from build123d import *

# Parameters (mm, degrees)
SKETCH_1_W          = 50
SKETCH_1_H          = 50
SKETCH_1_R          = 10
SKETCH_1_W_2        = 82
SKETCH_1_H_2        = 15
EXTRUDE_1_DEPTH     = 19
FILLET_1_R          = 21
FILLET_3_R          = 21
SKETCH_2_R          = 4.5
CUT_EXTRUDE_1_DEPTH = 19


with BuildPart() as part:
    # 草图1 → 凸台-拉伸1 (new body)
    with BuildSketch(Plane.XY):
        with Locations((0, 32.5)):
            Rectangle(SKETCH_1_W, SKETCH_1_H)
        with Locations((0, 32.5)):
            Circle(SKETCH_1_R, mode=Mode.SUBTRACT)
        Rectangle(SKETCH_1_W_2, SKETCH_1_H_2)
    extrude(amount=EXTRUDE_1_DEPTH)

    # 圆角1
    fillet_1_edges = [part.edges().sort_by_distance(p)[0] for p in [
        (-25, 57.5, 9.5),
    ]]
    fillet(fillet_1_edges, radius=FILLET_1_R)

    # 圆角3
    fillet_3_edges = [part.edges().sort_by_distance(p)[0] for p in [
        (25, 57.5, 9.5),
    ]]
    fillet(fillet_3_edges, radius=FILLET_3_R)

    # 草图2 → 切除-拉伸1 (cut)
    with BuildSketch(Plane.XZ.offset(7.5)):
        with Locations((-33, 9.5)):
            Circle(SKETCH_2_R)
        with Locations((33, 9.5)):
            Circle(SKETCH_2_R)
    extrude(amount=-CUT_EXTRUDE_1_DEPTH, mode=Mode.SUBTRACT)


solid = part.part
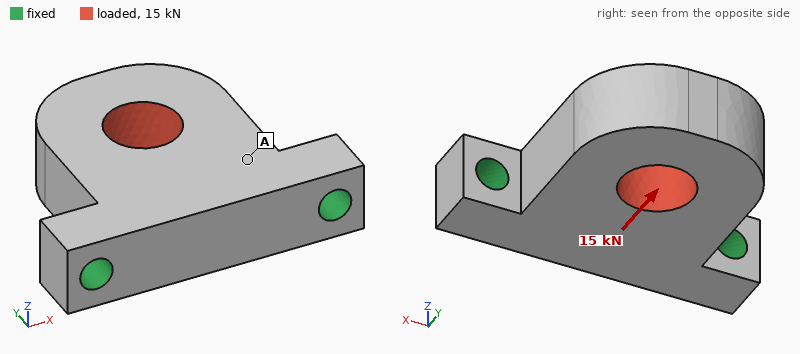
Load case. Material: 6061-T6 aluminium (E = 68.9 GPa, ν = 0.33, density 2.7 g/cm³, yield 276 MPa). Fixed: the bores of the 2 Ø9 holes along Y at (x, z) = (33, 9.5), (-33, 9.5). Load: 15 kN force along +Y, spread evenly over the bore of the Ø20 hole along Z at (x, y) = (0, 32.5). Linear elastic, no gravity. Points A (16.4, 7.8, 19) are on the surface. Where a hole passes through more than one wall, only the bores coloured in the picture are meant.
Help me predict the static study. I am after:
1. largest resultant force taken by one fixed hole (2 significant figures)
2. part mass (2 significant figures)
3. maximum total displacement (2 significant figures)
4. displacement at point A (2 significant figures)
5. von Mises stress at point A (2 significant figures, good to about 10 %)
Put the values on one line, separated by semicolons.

8.0 kN; 160 g; 28 µm; 16 µm; 20 MPa
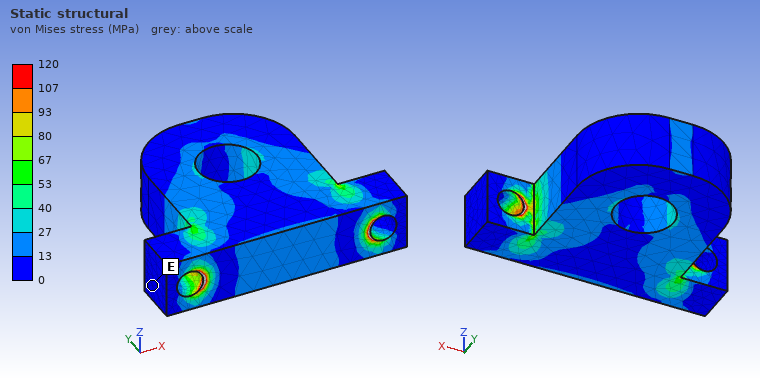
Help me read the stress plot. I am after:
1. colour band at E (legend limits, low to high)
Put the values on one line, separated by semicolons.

0 to 13 MPa
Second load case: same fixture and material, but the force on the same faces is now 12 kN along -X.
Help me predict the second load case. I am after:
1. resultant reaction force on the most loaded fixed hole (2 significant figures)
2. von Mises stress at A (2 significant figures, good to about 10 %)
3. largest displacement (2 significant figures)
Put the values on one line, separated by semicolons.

9.2 kN; 24 MPa; 67 µm
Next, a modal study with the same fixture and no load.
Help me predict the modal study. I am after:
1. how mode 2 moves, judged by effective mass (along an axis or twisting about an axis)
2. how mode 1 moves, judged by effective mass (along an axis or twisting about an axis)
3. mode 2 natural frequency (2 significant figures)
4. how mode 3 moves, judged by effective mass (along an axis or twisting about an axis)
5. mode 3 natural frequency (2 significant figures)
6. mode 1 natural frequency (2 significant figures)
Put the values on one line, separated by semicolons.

along X; along Z; 7800 Hz; twisting about Y; 9400 Hz; 2900 Hz
